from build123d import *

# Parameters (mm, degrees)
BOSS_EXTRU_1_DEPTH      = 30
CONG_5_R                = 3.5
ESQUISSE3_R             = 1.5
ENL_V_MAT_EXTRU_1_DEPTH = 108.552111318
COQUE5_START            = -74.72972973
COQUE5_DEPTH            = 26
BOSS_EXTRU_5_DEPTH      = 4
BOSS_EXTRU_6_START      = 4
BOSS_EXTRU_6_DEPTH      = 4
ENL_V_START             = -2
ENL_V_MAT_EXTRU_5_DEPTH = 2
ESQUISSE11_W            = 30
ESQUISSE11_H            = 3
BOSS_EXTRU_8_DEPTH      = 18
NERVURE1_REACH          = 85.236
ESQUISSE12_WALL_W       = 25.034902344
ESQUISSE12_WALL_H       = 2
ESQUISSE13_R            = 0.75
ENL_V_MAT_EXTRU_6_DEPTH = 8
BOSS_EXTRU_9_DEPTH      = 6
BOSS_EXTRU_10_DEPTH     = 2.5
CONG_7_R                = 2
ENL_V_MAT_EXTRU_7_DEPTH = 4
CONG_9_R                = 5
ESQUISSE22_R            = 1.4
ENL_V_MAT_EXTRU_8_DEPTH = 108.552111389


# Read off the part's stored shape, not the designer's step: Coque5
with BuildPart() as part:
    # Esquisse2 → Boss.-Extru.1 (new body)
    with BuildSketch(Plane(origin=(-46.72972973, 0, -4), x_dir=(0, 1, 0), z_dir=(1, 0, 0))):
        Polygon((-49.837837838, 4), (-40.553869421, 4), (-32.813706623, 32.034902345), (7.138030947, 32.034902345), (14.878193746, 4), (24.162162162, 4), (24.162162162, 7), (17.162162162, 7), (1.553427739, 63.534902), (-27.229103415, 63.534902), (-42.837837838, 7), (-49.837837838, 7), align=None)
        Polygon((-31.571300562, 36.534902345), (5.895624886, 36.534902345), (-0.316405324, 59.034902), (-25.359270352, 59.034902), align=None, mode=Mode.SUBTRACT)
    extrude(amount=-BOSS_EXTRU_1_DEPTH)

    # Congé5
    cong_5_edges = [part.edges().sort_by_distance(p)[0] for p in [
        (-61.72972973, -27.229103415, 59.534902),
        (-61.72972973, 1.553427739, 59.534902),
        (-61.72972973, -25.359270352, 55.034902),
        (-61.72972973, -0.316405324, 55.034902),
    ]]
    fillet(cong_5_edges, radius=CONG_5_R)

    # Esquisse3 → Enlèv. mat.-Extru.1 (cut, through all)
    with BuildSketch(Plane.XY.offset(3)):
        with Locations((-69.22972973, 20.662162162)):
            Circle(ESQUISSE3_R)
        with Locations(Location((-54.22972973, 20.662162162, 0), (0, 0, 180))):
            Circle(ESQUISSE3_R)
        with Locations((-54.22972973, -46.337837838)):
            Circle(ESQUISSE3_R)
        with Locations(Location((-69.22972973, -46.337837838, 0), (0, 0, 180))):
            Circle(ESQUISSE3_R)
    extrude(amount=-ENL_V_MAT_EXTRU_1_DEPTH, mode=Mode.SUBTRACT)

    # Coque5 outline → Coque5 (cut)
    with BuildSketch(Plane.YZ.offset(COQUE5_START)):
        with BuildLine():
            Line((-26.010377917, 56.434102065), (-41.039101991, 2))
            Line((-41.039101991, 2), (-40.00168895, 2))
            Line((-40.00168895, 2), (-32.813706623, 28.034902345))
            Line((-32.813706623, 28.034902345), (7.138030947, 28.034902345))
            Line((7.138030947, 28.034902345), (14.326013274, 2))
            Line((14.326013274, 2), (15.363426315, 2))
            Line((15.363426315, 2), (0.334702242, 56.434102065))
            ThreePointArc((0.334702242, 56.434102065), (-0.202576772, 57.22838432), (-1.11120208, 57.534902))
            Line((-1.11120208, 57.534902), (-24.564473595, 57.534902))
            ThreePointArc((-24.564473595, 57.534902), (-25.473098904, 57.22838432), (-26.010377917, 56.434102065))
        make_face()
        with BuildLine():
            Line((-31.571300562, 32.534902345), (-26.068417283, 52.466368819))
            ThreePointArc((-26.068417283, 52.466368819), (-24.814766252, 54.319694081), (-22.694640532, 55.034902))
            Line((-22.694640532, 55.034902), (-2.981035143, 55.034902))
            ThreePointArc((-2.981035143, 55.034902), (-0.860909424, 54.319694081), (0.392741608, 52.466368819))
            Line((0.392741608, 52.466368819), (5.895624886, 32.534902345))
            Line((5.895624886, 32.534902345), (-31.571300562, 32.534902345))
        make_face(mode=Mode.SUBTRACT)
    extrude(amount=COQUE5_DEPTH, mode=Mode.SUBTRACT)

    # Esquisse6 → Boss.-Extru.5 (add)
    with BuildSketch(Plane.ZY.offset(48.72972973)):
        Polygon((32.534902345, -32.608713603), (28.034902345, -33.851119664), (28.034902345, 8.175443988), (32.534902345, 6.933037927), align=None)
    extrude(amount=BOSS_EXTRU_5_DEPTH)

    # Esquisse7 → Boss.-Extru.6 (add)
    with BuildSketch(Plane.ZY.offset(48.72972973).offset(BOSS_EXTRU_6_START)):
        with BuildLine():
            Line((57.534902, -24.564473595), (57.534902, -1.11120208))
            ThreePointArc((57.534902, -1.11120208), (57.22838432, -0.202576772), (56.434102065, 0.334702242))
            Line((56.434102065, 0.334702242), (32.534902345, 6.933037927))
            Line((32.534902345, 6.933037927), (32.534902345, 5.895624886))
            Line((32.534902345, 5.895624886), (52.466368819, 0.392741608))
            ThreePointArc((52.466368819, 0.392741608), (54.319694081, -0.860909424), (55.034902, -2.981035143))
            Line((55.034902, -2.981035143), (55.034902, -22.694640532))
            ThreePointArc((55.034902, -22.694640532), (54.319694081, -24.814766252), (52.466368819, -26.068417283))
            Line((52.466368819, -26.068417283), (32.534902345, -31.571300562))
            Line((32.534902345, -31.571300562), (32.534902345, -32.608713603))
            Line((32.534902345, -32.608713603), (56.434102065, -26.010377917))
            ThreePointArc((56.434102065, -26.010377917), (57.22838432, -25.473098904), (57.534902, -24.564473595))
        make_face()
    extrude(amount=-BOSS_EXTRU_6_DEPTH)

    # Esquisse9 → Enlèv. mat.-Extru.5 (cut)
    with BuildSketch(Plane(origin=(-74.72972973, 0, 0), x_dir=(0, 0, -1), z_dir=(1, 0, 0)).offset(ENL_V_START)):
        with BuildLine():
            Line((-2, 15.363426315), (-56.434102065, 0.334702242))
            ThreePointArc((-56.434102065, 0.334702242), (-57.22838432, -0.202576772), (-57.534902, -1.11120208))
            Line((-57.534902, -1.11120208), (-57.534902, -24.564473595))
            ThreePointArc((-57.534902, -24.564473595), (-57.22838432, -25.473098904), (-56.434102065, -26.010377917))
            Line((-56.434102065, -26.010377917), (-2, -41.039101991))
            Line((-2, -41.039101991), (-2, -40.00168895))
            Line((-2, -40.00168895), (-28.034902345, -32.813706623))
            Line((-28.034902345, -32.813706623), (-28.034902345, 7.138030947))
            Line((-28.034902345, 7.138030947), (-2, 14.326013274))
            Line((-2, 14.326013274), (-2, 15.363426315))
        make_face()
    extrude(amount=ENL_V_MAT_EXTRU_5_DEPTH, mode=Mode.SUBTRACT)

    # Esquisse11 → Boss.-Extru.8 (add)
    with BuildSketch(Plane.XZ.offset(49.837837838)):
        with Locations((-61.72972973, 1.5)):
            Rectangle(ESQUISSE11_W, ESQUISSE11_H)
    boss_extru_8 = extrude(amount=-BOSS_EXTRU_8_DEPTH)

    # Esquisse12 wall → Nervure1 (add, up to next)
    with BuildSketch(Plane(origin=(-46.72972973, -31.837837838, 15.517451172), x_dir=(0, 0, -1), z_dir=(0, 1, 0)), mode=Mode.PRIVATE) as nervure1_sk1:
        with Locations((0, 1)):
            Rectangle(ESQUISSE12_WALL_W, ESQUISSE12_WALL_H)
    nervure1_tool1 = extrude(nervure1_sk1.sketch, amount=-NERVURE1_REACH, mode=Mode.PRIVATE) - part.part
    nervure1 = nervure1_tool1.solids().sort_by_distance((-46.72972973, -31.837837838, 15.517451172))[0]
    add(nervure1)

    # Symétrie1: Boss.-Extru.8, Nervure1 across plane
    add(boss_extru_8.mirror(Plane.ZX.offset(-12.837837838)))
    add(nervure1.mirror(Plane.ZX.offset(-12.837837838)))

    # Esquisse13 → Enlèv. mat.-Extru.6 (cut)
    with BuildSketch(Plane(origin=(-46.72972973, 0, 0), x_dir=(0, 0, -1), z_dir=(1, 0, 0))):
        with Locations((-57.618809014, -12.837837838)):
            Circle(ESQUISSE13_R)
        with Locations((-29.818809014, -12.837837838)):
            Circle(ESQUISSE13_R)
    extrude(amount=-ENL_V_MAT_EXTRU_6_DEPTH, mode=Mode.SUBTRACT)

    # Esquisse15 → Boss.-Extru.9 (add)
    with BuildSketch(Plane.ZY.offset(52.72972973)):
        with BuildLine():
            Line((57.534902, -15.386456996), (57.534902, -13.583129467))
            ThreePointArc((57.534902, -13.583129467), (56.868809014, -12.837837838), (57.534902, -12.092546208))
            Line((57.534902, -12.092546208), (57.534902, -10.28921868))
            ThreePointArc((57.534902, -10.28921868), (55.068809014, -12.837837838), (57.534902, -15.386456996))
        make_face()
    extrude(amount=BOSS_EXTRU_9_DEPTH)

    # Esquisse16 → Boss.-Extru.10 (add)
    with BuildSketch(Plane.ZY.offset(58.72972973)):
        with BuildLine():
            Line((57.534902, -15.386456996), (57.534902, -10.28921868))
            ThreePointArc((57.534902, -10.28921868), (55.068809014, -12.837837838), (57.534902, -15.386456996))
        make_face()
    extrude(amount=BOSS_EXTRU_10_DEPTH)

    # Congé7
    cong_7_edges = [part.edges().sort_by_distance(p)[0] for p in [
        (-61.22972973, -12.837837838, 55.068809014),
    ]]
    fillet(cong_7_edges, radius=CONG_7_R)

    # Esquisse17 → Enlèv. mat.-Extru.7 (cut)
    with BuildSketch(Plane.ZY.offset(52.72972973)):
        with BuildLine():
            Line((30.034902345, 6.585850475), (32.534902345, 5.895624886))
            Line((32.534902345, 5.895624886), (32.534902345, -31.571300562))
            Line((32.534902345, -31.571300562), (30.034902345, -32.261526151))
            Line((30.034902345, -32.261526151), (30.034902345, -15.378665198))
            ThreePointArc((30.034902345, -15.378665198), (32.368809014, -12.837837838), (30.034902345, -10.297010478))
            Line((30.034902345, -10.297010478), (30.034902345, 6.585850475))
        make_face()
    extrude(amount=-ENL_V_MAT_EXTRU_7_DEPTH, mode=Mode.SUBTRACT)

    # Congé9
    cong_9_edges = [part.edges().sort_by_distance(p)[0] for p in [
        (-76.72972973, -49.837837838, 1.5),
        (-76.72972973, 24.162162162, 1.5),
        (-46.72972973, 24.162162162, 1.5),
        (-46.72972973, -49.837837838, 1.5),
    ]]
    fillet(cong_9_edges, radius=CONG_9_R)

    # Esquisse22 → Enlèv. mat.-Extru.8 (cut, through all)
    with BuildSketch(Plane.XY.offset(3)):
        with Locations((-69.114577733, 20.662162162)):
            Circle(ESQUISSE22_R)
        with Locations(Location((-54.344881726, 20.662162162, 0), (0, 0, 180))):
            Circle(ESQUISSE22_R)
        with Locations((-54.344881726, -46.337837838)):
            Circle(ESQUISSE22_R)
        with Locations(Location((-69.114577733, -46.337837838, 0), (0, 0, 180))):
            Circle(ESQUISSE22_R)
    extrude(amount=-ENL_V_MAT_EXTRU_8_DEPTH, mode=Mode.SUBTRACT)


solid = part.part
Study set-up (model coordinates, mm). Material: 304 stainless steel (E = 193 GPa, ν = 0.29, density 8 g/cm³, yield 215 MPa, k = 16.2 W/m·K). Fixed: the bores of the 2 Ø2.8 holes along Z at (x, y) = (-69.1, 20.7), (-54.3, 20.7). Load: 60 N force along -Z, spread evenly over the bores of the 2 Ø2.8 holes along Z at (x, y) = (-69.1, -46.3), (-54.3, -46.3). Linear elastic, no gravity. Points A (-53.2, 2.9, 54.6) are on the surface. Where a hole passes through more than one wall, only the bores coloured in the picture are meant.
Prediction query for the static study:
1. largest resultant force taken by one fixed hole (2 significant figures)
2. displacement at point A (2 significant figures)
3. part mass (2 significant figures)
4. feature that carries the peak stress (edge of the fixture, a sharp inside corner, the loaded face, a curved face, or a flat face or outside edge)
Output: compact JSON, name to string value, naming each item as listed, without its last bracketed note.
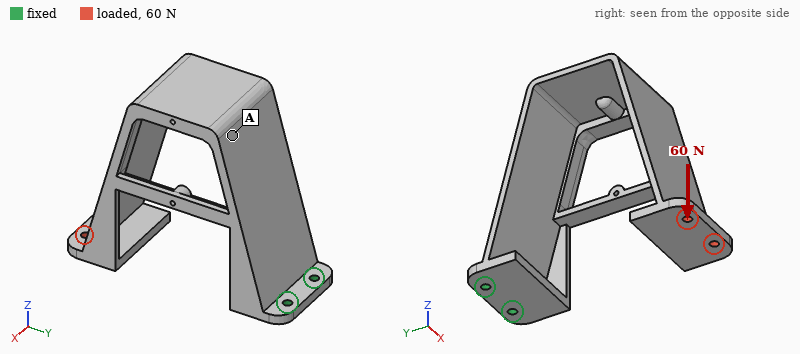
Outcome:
{"largest resultant force taken by one fixed hole": "75 N", "displacement at point A": "0.43 mm", "part mass": "110 g", "feature that carries the peak stress": "a flat face or outside edge"}
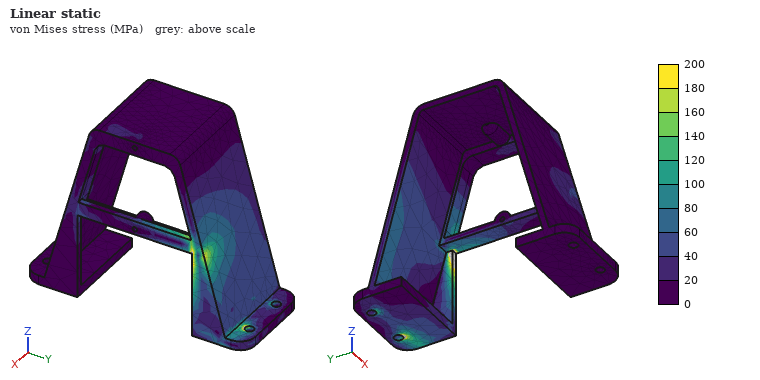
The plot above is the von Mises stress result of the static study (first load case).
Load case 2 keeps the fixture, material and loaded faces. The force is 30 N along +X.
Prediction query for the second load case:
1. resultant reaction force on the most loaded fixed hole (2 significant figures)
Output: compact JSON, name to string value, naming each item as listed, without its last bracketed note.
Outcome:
{"resultant reaction force on the most loaded fixed hole": "120 N"}
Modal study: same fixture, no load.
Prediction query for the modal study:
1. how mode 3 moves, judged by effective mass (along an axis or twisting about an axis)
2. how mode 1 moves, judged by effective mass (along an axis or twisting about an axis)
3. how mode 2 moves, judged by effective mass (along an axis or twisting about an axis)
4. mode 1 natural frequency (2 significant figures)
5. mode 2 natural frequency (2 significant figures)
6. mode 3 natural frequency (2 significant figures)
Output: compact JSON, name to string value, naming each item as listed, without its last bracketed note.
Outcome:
{"how mode 3 moves, judged by effective mass": "along Y", "how mode 1 moves, judged by effective mass": "along Z", "how mode 2 moves, judged by effective mass": "along X", "mode 1 natural frequency": "200 Hz", "mode 2 natural frequency": "250 Hz", "mode 3 natural frequency": "660 Hz"}
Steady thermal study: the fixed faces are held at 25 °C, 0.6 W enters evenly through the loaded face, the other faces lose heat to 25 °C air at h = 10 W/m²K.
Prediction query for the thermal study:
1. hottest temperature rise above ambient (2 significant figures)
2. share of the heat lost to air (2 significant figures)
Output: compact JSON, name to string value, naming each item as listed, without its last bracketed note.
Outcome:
{"hottest temperature rise above ambient": "17 K", "share of the heat lost to air": "95 %"}
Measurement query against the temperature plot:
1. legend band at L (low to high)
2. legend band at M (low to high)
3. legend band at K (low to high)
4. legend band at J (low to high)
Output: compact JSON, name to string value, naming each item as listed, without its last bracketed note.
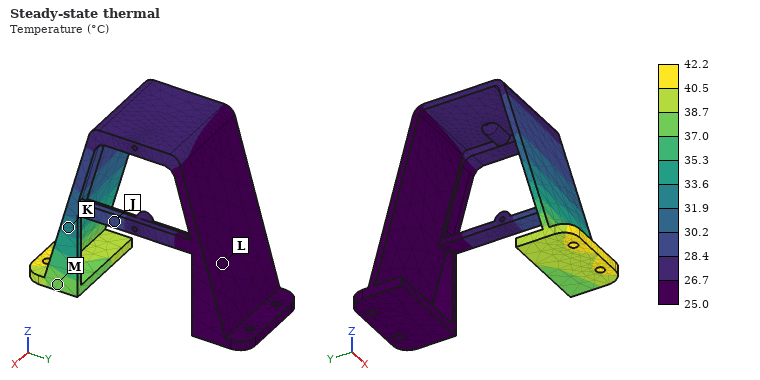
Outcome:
{"legend band at L": "25.0 to 26.7 °C", "legend band at M": "37.0 to 38.7 °C", "legend band at K": "31.9 to 33.6 °C", "legend band at J": "28.4 to 30.2 °C"}
